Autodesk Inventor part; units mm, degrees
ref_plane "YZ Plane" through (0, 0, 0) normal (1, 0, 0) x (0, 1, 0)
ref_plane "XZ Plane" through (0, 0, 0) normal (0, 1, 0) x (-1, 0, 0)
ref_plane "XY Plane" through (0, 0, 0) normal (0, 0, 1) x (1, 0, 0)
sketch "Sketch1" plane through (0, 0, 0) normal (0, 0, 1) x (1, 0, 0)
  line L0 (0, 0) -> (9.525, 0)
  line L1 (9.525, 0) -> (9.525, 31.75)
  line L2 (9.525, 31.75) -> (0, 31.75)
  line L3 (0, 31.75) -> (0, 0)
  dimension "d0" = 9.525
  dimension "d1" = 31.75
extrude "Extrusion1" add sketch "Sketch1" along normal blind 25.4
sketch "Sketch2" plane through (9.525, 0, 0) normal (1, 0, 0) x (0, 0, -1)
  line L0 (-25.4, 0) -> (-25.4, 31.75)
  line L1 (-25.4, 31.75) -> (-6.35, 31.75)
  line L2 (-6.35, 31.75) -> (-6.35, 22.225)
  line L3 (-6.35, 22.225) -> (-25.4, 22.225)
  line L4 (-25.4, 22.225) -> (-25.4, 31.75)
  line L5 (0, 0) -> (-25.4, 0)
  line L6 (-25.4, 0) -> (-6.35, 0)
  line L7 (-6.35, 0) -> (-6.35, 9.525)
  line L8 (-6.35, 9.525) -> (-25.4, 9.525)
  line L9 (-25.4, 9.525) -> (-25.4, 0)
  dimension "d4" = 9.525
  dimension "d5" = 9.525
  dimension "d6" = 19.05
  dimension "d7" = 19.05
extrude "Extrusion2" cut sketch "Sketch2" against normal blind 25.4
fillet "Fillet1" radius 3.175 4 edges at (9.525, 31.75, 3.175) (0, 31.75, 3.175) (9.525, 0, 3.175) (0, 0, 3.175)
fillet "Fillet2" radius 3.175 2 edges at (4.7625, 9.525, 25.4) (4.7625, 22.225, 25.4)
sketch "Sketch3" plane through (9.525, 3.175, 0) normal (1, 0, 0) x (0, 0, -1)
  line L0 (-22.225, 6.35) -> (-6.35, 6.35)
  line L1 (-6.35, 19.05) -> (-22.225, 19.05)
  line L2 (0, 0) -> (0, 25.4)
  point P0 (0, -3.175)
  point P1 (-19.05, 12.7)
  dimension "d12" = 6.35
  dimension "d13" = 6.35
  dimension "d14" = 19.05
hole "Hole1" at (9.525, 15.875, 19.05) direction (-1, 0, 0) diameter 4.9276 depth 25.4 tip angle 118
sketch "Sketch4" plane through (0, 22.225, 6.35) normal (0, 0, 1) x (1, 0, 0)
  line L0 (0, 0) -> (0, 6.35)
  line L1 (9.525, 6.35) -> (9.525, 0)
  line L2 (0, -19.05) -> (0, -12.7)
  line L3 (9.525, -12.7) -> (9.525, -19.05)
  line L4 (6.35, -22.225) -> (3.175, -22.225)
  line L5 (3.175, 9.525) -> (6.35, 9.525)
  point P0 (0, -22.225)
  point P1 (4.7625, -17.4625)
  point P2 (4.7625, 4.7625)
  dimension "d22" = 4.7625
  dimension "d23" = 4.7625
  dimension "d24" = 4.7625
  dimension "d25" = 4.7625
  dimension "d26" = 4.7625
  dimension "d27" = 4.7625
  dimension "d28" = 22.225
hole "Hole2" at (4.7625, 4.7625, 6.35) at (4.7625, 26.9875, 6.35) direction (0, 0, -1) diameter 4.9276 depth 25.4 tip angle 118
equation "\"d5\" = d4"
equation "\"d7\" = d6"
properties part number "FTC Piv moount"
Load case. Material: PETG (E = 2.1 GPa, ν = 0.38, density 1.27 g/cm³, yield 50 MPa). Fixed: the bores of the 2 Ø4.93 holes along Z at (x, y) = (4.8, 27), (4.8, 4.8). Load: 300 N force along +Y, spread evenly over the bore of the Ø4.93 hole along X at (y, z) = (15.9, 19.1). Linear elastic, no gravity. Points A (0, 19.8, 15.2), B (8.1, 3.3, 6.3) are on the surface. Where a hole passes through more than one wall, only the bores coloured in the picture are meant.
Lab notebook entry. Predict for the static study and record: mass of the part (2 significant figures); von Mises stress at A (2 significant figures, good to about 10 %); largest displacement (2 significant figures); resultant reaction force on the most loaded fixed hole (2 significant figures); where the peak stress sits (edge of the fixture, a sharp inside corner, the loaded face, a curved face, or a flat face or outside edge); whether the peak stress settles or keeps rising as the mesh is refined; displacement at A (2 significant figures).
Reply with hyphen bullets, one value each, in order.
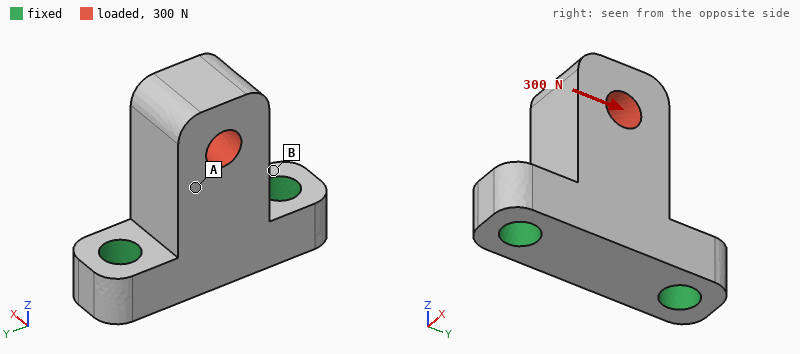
- 4.7 g
- 4.3 MPa
- 0.30 mm
- 320 N
- a sharp inside corner
- keeps rising
- 0.14 mm
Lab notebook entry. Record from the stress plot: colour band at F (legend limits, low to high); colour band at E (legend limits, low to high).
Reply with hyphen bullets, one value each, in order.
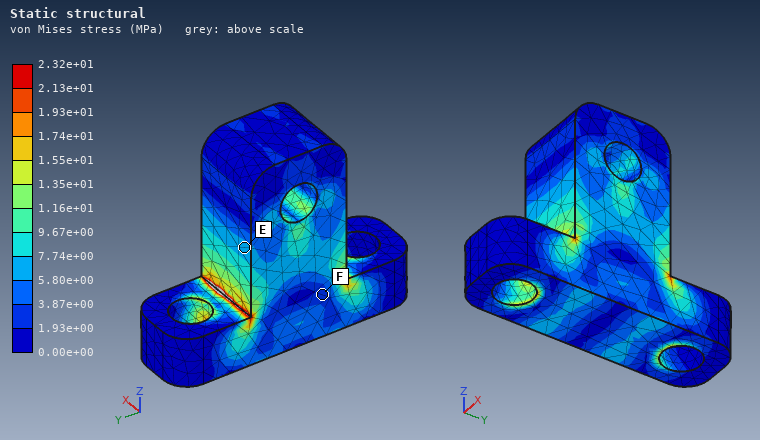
- 1.93e+00 to 3.87e+00 MPa
- 5.80e+00 to 7.74e+00 MPa
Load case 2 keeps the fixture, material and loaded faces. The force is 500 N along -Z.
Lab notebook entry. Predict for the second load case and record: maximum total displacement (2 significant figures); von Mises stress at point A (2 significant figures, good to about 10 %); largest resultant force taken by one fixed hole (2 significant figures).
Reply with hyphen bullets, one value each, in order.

- 82 µm
- 5.0 MPa
- 260 N
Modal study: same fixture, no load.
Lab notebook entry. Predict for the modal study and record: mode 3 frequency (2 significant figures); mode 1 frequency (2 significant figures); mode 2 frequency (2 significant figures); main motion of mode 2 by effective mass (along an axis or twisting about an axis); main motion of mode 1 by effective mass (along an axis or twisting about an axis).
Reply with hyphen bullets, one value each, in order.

- 8000 Hz
- 2400 Hz
- 4300 Hz
- along Y
- along X
